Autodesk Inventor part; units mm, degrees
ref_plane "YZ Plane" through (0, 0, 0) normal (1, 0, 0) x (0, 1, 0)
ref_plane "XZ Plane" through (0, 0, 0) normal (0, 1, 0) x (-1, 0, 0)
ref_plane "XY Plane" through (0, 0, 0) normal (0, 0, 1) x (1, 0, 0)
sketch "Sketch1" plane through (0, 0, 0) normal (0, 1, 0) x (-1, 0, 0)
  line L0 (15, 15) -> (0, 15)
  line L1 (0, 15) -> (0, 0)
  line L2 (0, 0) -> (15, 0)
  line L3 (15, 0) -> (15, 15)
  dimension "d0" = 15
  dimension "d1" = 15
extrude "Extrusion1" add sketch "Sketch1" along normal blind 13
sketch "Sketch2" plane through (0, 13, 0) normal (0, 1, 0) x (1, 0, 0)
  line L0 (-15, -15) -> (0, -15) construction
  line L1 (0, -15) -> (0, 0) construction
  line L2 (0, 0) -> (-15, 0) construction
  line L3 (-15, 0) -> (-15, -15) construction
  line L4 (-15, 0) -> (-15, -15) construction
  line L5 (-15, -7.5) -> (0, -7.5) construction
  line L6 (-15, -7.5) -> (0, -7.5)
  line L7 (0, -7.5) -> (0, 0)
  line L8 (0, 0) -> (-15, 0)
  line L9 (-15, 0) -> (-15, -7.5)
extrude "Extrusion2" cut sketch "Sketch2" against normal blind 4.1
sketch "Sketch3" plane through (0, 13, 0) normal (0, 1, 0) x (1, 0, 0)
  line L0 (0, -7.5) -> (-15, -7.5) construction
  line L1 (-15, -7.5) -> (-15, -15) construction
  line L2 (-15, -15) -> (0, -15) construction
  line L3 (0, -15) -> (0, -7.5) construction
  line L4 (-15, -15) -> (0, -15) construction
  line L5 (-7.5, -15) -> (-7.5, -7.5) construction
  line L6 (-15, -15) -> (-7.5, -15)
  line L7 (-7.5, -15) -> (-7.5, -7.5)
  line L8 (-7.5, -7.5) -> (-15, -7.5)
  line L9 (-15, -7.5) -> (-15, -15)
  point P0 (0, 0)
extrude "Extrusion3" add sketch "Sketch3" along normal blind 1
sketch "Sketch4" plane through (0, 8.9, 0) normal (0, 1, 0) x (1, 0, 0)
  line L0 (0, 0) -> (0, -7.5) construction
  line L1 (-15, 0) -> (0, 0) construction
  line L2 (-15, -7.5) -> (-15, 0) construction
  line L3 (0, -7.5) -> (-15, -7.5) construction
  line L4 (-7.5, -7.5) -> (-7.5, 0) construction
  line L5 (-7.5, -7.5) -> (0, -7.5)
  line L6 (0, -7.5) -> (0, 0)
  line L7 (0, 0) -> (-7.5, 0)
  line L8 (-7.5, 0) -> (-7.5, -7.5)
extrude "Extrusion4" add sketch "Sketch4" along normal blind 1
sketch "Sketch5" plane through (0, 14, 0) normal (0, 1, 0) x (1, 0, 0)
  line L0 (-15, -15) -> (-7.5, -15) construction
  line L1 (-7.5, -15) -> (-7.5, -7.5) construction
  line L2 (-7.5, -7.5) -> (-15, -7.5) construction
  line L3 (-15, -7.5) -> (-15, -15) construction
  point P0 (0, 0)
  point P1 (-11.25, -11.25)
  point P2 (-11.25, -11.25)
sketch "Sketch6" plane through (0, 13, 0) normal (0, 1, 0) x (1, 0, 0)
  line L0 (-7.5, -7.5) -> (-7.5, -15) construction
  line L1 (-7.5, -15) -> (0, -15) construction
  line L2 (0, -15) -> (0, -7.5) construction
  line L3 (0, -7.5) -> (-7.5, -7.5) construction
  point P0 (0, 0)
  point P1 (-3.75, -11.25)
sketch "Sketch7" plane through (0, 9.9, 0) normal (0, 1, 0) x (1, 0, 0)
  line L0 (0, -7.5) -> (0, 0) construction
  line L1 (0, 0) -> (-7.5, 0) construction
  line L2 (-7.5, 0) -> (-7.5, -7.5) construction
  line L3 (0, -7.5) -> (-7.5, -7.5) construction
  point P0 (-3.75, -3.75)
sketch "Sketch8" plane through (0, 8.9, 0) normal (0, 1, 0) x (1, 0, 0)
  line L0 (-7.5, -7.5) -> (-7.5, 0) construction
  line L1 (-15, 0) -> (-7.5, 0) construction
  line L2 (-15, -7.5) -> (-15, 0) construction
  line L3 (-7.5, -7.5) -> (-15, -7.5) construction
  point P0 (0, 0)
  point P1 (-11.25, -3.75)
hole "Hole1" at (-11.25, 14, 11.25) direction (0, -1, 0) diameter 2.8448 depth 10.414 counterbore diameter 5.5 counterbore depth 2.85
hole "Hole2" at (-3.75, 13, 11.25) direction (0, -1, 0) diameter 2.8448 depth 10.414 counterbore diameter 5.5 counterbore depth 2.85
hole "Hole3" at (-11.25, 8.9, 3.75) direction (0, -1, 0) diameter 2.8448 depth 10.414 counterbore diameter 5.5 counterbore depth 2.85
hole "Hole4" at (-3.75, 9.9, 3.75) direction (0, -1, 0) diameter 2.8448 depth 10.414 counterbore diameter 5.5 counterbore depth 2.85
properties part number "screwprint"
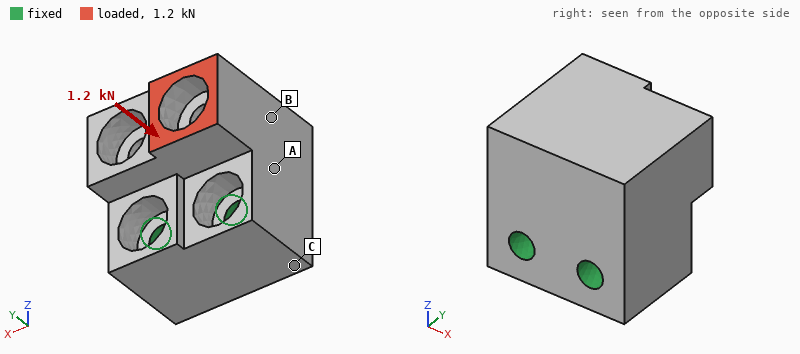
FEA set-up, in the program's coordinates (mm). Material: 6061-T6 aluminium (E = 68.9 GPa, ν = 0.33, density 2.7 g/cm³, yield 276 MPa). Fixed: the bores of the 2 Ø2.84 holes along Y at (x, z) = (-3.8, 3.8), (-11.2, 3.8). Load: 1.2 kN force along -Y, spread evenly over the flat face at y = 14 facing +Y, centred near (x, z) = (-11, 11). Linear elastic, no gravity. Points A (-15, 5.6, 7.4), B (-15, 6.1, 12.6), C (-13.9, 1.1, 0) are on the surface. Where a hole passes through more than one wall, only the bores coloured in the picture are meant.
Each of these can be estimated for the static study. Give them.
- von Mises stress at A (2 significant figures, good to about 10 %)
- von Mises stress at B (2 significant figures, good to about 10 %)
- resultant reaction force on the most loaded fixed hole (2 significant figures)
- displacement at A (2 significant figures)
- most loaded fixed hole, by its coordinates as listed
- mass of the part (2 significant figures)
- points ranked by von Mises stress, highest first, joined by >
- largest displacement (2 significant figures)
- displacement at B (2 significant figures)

45 MPa
25 MPa
930 N
6.4 µm
(-11.2, 3.8)
5.7 g
A > B > C
27 µm
15 µm
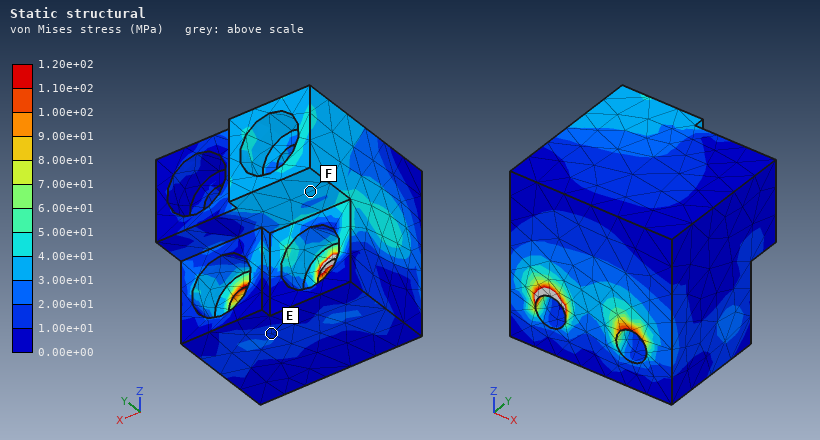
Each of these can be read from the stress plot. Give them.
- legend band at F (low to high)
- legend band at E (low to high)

3.00e+01 to 4.00e+01 MPa
1.00e+01 to 2.00e+01 MPa
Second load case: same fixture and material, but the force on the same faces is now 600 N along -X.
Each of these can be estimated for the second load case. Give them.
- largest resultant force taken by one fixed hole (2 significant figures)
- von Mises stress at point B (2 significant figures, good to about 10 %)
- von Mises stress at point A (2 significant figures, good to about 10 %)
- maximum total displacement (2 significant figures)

770 N
17 MPa
31 MPa
21 µm
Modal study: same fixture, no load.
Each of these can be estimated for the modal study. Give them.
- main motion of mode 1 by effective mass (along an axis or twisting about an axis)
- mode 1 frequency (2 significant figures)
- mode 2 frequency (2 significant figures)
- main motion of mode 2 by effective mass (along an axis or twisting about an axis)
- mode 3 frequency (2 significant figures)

along Y
26 kHz
36 kHz
along X
45 kHz
